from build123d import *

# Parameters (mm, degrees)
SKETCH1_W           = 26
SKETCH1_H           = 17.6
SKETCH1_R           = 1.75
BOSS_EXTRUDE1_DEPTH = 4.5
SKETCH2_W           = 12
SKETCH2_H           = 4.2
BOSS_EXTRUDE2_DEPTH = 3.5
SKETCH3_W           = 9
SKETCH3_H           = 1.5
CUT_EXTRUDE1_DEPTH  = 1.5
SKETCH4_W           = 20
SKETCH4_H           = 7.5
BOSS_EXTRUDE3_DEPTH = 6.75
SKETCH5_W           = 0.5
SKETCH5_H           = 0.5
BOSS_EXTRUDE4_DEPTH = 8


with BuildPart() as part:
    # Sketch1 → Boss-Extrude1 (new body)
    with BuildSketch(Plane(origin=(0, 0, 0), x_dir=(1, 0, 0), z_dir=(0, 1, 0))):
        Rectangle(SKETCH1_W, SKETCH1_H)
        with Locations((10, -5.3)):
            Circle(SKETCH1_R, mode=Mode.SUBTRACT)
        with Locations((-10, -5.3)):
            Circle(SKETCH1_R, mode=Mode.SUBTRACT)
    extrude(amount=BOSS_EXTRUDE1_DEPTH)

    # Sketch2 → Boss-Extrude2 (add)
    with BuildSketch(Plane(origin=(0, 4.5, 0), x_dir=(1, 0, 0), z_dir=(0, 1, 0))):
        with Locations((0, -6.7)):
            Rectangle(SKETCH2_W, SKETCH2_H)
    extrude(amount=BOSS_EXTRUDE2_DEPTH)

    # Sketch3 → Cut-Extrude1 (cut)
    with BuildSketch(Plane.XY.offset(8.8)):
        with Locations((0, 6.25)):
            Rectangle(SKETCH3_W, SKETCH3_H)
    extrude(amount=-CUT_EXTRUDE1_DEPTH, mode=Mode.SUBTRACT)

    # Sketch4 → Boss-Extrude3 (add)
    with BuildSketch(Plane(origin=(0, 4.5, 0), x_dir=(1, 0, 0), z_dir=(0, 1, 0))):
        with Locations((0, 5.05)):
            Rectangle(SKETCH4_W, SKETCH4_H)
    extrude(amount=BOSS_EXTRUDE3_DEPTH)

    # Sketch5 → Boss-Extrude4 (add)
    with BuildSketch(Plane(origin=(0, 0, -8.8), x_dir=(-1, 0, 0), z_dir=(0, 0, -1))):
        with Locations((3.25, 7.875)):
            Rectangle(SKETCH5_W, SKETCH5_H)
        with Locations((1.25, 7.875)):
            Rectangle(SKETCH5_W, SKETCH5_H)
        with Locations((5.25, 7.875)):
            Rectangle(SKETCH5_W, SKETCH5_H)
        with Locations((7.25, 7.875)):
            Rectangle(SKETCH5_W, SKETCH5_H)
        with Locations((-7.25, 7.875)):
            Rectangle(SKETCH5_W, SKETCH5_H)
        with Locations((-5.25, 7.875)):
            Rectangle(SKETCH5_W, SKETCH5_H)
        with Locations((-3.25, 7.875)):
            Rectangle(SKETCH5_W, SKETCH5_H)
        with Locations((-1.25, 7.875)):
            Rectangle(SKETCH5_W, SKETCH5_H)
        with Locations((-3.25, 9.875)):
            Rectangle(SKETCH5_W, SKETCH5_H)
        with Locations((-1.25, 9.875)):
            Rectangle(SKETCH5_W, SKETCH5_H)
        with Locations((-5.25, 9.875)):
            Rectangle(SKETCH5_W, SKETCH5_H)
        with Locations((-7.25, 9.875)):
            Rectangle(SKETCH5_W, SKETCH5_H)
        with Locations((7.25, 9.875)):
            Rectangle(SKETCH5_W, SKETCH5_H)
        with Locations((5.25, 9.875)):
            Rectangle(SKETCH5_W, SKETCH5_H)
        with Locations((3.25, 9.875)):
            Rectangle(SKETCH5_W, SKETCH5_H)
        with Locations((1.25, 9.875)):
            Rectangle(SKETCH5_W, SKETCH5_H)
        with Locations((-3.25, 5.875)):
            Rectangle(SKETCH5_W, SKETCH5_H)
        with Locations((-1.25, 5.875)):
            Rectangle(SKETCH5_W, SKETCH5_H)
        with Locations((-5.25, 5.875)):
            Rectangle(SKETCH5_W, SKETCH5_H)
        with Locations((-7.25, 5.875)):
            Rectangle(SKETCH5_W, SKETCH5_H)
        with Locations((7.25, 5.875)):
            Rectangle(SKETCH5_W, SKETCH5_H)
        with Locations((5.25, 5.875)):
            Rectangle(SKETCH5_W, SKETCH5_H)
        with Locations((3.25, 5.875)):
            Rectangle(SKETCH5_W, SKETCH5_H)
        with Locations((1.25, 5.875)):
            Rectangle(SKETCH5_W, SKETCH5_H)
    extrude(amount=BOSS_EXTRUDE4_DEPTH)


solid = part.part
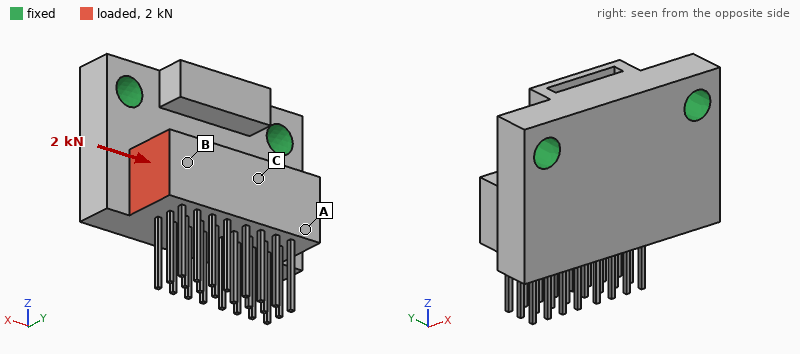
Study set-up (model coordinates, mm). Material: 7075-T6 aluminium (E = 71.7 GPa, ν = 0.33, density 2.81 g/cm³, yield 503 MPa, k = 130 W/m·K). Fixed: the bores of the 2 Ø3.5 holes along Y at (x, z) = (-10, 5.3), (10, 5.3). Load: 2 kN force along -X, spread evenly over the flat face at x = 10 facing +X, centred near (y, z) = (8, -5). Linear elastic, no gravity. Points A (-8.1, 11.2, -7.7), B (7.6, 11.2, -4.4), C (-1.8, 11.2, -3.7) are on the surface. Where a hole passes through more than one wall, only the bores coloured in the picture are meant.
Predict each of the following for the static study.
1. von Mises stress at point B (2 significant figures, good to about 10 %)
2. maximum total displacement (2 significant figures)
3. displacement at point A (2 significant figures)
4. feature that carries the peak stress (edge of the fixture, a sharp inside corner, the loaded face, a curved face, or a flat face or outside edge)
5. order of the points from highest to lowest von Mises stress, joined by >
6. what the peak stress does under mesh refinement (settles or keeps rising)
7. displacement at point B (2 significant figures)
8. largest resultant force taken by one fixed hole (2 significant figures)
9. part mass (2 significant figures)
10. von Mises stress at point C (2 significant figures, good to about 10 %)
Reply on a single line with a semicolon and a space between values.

43 MPa; 28 µm; 22 µm; edge of the fixture; B > C > A; keeps rising; 25 µm; 1.5 kN; 9.0 g; 24 MPa
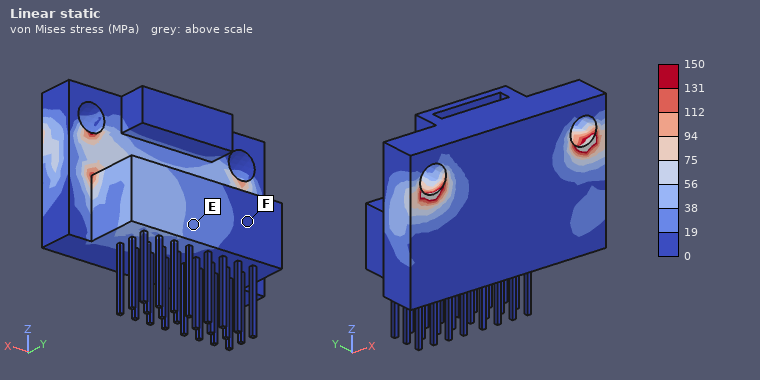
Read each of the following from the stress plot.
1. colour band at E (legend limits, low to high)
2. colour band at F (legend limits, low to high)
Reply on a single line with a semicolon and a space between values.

19 to 38 MPa; 0 to 19 MPa
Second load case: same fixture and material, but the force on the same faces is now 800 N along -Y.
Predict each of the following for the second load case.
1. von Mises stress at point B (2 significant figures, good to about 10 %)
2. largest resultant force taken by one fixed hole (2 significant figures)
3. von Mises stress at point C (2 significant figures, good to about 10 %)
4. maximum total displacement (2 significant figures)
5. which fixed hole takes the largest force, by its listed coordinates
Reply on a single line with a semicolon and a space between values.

25 MPa; 810 N; 13 MPa; 78 µm; (10, 5.3)
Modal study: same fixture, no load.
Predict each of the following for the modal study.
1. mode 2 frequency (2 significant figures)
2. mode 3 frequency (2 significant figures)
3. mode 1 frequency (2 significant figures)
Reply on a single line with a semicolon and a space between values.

6200 Hz; 6200 Hz; 6200 Hz
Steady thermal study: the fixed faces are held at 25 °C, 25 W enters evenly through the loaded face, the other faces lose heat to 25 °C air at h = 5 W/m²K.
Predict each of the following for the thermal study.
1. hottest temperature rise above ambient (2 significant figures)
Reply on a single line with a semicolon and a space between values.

40 K
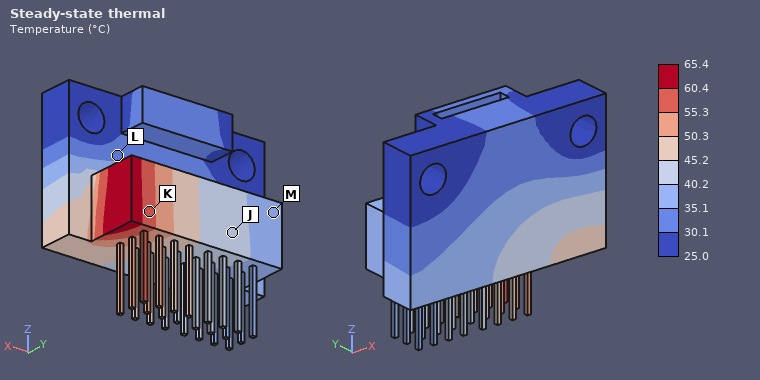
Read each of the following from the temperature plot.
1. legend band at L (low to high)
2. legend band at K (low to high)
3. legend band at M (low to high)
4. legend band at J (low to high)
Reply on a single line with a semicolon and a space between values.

30.1 to 35.1 °C; 55.3 to 60.4 °C; 35.1 to 40.2 °C; 40.2 to 45.2 °C
